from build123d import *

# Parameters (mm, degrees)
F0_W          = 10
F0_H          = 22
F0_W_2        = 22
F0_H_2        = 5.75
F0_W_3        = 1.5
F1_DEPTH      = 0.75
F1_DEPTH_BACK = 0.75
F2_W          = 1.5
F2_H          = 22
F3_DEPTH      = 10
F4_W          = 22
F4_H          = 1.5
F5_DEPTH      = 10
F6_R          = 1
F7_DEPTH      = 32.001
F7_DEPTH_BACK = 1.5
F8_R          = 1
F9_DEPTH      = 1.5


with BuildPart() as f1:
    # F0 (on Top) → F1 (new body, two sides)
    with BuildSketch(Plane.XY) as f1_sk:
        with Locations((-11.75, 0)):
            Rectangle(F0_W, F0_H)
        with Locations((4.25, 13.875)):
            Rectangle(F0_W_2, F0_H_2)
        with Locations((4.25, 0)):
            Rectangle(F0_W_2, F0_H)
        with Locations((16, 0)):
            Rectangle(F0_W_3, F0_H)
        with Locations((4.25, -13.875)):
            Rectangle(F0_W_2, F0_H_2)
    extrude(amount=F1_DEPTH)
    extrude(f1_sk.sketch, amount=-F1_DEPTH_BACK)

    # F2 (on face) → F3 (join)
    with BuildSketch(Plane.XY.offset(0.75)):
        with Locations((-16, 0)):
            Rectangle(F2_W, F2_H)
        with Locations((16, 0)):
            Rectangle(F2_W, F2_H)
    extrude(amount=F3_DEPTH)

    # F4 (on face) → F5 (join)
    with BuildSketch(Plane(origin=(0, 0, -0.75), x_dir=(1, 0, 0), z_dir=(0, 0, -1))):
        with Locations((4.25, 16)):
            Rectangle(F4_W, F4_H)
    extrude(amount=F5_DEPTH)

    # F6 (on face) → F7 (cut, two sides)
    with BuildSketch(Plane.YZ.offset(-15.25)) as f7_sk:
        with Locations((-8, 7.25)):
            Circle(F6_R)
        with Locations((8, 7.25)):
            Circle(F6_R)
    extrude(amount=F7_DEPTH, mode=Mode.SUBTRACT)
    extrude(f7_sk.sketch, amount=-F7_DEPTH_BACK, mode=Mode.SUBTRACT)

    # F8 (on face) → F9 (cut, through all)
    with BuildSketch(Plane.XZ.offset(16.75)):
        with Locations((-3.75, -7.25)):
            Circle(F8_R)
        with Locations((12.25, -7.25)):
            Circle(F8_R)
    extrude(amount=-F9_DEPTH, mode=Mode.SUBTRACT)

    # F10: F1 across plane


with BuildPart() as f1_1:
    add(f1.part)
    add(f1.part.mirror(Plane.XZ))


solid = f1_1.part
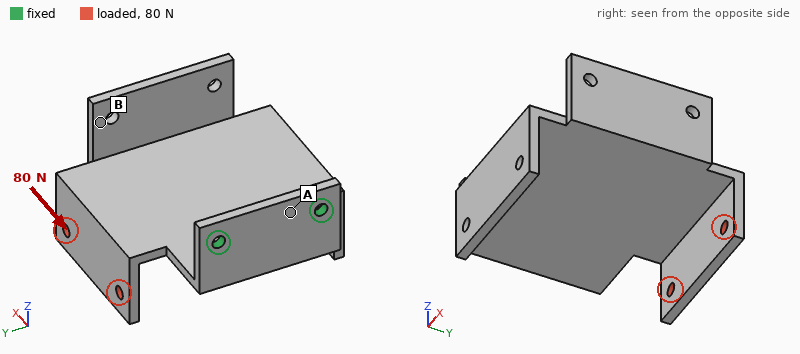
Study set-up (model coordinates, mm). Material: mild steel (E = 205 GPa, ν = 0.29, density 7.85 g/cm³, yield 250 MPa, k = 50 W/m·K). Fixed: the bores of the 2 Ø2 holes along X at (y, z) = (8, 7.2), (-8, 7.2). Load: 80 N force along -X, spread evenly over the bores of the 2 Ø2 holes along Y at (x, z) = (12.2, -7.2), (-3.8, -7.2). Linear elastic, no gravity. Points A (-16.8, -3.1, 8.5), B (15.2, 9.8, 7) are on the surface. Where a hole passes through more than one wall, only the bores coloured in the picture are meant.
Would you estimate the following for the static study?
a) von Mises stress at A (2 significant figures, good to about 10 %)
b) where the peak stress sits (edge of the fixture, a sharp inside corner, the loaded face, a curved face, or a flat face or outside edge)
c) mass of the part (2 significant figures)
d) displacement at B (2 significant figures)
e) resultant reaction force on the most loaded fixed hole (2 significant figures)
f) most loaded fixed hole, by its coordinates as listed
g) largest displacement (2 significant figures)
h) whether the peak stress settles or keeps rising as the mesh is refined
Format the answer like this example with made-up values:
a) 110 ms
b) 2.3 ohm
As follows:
a) 37 MPa
b) edge of the fixture
c) 22 g
d) 0.35 mm
e) 120 N
f) (8, 7.2)
g) 0.41 mm
h) keeps rising
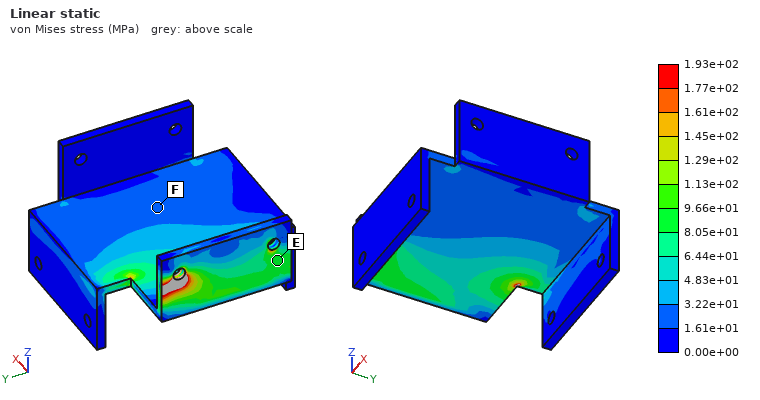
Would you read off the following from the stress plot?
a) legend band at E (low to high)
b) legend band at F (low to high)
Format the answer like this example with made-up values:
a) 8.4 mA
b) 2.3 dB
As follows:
a) 8.05e+01 to 9.66e+01 MPa
b) 1.61e+01 to 3.22e+01 MPa
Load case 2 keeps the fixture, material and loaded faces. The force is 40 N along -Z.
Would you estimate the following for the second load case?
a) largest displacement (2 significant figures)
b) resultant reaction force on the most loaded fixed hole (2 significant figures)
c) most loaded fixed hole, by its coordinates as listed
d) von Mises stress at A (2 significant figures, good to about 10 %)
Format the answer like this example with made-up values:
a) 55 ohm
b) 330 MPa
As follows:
a) 0.39 mm
b) 59 N
c) (8, 7.2)
d) 28 MPa
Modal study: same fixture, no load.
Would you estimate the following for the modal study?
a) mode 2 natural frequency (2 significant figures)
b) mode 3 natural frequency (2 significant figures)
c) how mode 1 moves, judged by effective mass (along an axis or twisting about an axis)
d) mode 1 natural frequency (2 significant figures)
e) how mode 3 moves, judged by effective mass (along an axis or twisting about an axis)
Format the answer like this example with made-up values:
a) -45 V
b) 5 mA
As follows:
a) 1200 Hz
b) 1700 Hz
c) along Z
d) 480 Hz
e) along Y
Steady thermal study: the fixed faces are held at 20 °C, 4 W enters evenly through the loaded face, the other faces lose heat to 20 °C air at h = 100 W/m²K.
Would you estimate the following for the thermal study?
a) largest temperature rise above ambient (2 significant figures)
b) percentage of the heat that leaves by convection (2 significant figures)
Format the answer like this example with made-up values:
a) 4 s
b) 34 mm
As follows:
a) 40 K
b) 88 %
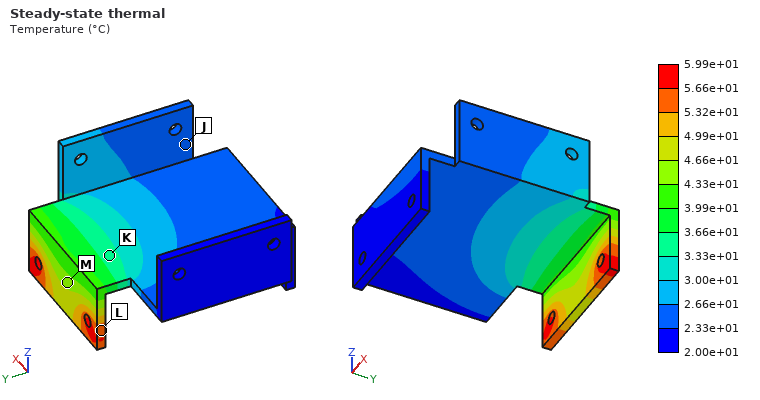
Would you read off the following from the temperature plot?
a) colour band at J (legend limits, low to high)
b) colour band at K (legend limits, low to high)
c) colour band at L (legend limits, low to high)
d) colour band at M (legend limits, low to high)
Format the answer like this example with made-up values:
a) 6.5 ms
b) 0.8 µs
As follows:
a) 2.33e+01 to 2.66e+01 °C
b) 3.33e+01 to 3.66e+01 °C
c) 5.32e+01 to 5.66e+01 °C
d) 4.33e+01 to 4.66e+01 °C
